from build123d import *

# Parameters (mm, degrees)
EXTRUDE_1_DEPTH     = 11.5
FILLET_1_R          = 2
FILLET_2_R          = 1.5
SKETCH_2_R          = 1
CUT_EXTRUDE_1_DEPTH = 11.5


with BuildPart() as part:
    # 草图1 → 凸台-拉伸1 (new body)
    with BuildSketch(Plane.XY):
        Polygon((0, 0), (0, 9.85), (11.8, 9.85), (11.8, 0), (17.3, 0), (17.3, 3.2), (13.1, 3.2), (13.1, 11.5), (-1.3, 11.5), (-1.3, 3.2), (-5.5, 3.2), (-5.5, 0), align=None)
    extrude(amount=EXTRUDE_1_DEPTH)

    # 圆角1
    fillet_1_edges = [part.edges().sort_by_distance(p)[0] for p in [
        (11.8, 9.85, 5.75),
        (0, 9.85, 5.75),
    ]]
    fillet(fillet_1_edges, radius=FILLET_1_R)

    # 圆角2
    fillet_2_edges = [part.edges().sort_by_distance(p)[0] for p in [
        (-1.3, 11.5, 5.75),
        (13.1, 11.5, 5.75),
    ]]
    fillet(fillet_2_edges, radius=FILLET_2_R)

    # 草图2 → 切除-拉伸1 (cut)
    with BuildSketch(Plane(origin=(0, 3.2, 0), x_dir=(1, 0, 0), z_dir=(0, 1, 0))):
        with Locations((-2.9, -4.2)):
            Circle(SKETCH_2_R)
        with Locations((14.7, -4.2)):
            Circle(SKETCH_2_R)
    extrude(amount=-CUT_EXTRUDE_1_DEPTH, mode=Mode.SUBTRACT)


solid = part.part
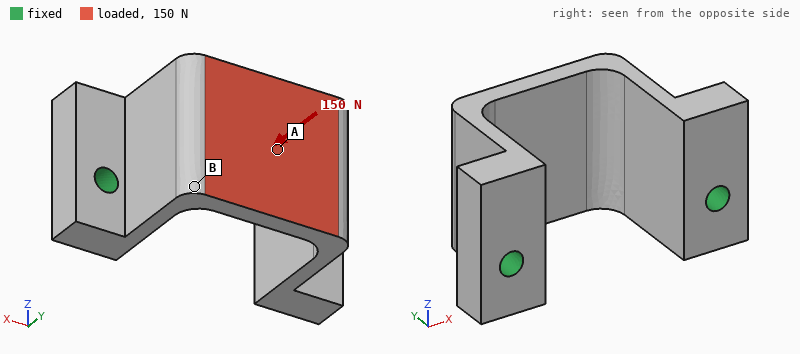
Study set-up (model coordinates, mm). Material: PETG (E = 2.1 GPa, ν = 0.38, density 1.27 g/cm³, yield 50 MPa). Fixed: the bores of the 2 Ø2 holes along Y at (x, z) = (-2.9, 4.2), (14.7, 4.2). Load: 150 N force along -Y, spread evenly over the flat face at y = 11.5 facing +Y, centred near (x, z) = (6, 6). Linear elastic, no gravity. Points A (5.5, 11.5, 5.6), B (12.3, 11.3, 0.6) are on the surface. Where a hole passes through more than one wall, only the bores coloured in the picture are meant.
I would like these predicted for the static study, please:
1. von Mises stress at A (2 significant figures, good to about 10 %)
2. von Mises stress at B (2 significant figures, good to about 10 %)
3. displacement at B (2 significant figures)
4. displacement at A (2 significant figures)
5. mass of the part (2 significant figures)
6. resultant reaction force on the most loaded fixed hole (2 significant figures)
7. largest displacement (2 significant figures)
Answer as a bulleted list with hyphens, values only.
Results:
- 20 MPa
- 3.7 MPa
- 0.056 mm
- 0.21 mm
- 1.1 g
- 80 N
- 0.27 mm
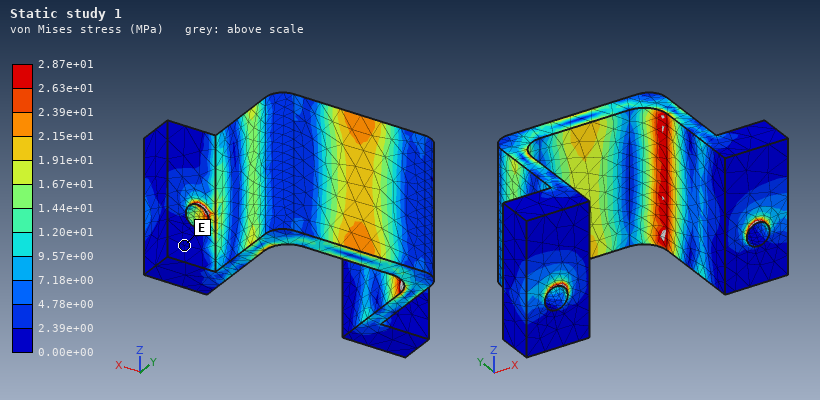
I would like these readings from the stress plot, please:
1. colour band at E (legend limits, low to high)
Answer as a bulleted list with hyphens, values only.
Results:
- 0.00e+00 to 2.39e+00 MPa
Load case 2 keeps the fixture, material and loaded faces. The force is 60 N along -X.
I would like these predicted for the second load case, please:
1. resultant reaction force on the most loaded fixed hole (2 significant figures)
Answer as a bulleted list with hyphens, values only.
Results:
- 39 N
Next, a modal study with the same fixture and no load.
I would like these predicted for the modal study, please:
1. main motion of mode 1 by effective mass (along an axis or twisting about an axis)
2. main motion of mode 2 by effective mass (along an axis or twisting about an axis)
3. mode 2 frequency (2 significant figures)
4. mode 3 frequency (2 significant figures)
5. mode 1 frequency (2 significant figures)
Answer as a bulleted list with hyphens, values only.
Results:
- along X
- along Z
- 4300 Hz
- 5800 Hz
- 3500 Hz
